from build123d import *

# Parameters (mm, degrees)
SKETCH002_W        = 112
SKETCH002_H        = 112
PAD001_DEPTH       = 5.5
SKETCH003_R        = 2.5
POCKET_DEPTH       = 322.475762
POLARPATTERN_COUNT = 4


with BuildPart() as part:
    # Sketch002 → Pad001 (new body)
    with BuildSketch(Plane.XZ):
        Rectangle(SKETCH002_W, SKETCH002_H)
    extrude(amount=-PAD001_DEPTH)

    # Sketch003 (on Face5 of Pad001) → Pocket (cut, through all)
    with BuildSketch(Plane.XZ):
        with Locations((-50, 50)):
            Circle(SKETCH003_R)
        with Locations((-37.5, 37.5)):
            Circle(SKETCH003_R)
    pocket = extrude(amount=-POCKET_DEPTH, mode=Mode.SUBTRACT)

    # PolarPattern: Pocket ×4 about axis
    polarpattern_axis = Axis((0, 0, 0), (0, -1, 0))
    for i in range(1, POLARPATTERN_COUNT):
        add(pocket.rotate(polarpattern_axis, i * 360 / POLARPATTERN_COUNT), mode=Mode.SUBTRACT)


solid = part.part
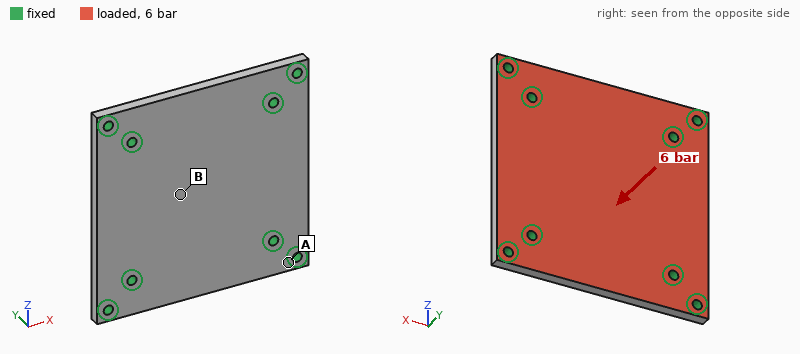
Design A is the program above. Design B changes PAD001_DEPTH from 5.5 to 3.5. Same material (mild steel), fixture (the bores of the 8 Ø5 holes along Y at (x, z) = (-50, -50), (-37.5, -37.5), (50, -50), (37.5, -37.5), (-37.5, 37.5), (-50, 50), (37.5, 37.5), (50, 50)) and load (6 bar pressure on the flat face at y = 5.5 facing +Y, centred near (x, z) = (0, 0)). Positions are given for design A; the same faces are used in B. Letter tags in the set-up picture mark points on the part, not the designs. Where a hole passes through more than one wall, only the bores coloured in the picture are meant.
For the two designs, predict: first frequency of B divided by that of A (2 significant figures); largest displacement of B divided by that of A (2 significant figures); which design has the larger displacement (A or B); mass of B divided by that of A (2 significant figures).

0.66
3.6
B
0.64
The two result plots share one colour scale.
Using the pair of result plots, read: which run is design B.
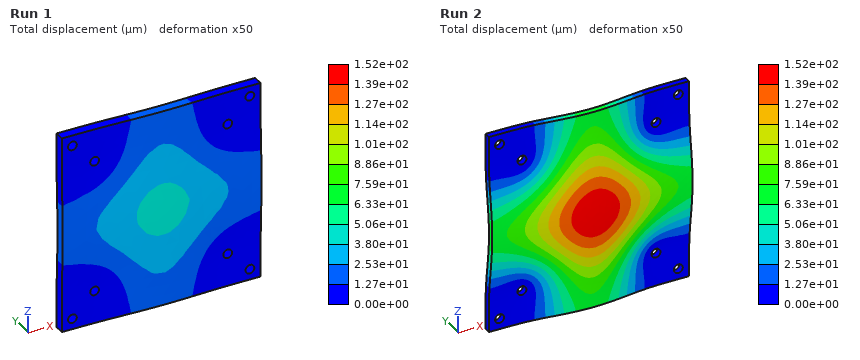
Run 2
